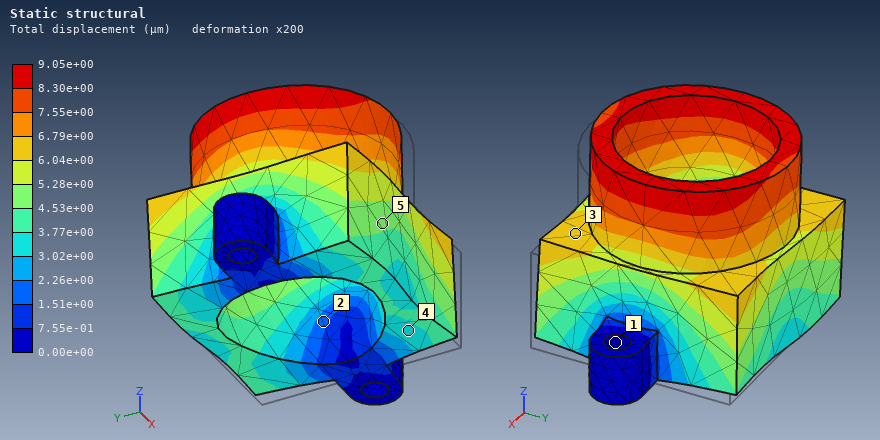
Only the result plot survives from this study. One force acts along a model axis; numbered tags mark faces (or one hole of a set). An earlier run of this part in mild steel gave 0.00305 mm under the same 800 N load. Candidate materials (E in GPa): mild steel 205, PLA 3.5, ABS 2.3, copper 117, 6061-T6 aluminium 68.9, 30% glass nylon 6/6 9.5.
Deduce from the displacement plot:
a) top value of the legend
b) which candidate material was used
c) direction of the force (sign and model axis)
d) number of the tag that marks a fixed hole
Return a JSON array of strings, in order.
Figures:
["9.05e+00 µm", "6061-T6 aluminium", "-X", "1"]
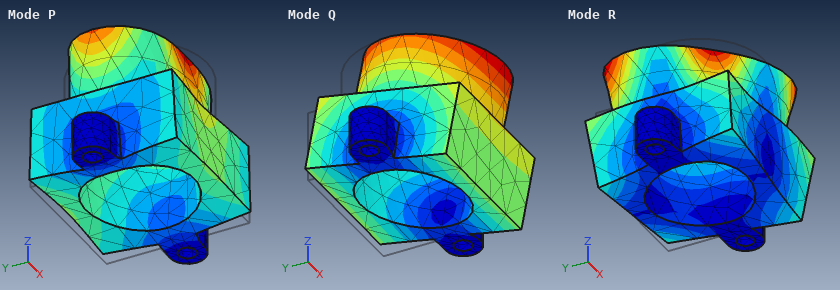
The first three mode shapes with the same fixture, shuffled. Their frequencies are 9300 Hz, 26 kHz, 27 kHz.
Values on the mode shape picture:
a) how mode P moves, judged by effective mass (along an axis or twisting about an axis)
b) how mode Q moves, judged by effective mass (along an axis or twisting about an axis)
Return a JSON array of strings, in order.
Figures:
["along Z", "along Y"]
